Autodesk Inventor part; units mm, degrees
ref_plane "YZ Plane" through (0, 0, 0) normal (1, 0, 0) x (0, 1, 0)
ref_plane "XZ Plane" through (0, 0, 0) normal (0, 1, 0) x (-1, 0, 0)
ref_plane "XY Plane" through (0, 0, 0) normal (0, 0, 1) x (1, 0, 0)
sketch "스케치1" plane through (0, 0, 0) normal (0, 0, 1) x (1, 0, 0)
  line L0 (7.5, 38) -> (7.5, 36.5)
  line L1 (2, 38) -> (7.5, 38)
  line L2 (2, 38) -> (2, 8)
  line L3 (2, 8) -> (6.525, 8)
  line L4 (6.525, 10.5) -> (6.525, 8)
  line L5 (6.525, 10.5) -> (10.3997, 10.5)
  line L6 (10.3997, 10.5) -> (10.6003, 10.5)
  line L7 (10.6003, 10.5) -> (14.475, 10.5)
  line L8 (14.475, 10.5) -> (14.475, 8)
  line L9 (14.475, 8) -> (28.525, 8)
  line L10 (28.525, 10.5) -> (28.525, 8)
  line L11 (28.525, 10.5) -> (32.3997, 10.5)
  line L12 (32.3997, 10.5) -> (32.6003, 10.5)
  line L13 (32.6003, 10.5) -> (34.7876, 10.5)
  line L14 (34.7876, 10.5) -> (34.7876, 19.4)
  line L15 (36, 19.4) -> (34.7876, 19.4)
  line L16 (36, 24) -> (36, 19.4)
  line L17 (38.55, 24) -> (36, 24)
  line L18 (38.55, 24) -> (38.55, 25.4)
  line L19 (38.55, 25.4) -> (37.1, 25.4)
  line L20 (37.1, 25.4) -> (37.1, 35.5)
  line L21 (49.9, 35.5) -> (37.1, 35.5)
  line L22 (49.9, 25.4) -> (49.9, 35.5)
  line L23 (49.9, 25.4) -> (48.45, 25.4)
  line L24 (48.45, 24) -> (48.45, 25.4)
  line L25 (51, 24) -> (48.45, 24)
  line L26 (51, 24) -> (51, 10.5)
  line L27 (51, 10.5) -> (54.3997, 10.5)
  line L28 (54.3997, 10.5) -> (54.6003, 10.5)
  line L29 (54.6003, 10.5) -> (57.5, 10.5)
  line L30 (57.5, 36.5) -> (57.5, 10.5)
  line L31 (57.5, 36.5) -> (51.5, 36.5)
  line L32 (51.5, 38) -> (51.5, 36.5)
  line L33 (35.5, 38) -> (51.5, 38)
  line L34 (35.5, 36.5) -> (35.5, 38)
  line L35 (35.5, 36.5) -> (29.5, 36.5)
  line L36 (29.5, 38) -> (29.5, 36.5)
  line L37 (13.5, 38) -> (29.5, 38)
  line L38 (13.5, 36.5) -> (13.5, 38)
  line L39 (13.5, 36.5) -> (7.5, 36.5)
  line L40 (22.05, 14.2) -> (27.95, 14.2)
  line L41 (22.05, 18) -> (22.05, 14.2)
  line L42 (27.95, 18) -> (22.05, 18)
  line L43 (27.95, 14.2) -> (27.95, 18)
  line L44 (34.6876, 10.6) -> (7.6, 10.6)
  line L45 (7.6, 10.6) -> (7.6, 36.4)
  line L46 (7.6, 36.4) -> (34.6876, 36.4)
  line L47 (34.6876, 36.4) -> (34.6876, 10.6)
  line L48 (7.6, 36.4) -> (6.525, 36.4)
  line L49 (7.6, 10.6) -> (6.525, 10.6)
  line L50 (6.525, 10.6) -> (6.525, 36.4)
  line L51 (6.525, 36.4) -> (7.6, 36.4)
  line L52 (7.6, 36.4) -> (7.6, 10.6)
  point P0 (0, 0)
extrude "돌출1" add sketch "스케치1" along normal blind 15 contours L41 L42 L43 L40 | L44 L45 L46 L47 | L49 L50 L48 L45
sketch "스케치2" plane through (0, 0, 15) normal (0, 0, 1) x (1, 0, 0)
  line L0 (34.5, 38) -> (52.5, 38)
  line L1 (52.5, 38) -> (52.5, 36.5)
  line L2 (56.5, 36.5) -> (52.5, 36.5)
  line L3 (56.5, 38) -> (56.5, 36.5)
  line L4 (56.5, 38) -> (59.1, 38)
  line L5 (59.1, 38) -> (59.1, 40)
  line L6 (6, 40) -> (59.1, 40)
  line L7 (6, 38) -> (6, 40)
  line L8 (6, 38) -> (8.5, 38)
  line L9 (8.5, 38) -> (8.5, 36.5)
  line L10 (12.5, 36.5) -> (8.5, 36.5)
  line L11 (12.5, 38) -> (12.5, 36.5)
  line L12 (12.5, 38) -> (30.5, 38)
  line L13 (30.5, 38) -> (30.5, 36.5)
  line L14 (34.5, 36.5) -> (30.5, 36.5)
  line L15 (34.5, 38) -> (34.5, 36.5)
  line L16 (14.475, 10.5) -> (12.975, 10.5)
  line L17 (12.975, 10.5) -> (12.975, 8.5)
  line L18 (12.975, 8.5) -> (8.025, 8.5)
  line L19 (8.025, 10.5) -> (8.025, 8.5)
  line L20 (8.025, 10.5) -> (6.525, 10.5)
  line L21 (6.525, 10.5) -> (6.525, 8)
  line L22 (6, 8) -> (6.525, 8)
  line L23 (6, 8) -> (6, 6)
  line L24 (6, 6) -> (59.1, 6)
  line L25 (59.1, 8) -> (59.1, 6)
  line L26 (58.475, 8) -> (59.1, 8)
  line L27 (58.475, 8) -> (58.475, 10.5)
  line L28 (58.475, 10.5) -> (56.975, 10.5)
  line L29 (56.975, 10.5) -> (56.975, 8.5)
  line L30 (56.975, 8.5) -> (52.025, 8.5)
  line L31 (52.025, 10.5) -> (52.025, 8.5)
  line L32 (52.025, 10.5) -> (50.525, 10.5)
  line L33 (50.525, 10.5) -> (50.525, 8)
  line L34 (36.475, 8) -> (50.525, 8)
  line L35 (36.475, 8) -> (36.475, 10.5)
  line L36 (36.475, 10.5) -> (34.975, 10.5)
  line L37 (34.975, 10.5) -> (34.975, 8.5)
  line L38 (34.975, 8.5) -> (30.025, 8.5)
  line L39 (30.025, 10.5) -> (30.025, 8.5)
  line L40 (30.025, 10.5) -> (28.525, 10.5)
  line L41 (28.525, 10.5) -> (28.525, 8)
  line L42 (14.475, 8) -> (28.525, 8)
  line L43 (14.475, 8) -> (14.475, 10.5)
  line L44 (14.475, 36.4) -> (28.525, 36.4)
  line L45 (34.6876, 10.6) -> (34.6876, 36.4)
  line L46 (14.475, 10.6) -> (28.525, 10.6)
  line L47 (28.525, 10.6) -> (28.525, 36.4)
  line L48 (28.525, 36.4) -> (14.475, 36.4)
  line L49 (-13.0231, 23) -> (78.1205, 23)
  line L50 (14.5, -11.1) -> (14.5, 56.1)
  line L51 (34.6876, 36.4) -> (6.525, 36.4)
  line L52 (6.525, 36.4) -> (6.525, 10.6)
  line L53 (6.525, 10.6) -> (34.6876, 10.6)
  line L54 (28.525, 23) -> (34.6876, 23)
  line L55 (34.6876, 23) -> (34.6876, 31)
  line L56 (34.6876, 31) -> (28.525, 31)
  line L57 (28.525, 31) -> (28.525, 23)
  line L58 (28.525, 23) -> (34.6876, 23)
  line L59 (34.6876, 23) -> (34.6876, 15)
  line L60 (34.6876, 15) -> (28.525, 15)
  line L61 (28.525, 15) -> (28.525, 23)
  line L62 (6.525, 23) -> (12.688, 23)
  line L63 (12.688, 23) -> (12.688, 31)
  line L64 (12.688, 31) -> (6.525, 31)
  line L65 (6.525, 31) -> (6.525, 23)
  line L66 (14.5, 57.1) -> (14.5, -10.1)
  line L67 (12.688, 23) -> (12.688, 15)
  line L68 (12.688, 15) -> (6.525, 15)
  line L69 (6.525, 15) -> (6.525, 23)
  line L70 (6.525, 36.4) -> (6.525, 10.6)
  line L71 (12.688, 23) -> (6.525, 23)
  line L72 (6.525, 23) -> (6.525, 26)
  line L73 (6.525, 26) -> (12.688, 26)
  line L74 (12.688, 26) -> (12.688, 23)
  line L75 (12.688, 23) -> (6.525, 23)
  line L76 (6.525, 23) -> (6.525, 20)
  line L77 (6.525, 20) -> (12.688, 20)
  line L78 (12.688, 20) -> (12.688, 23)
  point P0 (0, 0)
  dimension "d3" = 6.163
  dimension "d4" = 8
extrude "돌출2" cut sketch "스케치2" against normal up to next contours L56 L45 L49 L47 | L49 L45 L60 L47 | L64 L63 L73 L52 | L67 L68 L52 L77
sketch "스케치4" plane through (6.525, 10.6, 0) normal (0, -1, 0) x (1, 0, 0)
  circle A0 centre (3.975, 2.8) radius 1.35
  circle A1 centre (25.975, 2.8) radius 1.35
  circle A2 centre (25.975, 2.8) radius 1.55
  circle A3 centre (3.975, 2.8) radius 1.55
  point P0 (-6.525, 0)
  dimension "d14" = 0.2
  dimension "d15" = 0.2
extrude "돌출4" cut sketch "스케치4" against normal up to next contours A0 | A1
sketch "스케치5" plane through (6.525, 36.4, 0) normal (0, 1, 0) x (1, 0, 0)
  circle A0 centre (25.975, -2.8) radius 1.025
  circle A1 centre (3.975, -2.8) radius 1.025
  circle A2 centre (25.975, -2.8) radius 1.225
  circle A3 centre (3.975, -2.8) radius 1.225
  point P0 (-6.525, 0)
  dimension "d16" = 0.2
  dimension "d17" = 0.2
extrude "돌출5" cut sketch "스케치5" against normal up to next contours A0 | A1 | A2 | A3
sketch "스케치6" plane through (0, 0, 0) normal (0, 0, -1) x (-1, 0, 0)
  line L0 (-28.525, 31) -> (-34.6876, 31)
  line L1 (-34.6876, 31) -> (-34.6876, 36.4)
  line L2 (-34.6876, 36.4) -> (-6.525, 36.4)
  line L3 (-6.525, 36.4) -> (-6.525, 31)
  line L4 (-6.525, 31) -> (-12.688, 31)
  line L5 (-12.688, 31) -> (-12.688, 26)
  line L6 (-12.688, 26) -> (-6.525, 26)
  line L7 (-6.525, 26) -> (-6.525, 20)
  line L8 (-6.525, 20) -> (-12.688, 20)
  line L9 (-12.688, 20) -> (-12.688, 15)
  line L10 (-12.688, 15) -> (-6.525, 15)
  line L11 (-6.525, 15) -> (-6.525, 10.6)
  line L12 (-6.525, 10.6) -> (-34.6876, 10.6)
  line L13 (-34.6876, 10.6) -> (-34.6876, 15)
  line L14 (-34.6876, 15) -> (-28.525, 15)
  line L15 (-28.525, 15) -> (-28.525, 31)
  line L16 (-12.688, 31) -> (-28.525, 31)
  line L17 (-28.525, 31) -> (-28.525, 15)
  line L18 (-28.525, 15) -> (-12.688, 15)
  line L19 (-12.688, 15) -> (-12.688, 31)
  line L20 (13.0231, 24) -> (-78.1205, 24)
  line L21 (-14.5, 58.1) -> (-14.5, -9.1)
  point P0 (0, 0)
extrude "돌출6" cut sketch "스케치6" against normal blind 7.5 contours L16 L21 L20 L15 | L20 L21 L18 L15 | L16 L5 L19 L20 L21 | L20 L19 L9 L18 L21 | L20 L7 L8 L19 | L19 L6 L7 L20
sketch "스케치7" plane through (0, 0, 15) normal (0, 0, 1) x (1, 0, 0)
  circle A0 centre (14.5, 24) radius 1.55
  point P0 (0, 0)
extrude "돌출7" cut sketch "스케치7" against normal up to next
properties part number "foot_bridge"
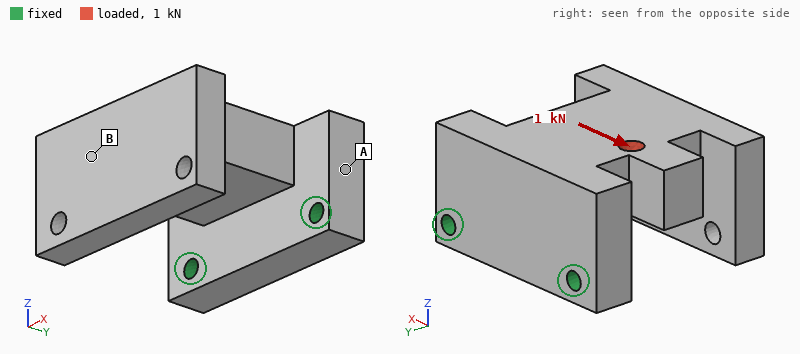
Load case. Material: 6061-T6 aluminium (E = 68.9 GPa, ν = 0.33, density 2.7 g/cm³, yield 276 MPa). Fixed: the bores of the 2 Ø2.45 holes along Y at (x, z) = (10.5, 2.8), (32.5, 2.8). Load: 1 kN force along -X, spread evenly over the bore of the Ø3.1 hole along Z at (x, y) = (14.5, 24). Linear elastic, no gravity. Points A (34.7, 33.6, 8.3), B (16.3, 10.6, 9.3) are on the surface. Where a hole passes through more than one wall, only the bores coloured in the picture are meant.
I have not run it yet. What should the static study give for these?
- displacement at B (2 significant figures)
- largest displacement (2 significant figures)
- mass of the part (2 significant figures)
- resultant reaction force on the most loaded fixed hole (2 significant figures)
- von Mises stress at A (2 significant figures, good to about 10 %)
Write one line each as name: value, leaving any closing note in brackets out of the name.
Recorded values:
displacement at B: 28 µm
largest displacement: 34 µm
mass of the part: 17 g
resultant reaction force on the most loaded fixed hole: 780 N
von Mises stress at A: 23 MPa
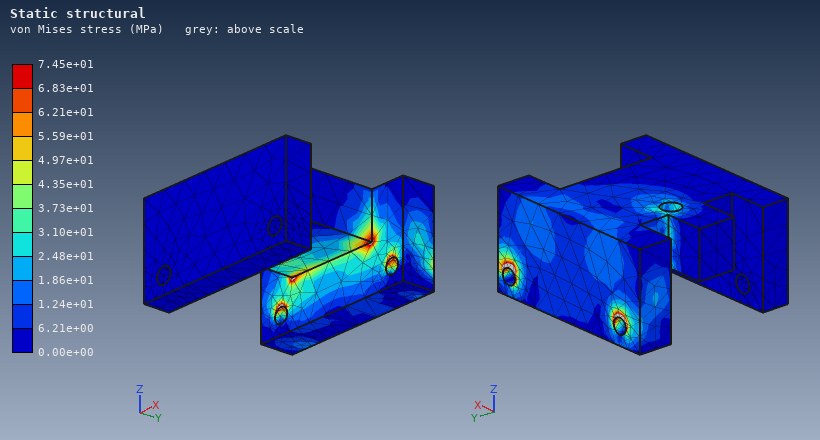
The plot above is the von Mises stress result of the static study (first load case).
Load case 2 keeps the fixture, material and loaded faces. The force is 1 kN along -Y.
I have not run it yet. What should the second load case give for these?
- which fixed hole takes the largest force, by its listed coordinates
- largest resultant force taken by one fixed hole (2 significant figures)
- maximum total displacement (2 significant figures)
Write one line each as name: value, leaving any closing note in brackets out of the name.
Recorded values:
which fixed hole takes the largest force, by its listed coordinates: (10.5, 2.8)
largest resultant force taken by one fixed hole: 830 N
maximum total displacement: 75 µm
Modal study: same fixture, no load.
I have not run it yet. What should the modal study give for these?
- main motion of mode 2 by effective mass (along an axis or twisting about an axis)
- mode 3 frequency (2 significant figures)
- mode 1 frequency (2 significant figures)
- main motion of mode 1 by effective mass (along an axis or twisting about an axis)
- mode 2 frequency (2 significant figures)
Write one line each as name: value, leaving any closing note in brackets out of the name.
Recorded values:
main motion of mode 2 by effective mass: along X
mode 3 frequency: 11 kHz
mode 1 frequency: 3700 Hz
main motion of mode 1 by effective mass: along Z
mode 2 frequency: 6800 Hz
